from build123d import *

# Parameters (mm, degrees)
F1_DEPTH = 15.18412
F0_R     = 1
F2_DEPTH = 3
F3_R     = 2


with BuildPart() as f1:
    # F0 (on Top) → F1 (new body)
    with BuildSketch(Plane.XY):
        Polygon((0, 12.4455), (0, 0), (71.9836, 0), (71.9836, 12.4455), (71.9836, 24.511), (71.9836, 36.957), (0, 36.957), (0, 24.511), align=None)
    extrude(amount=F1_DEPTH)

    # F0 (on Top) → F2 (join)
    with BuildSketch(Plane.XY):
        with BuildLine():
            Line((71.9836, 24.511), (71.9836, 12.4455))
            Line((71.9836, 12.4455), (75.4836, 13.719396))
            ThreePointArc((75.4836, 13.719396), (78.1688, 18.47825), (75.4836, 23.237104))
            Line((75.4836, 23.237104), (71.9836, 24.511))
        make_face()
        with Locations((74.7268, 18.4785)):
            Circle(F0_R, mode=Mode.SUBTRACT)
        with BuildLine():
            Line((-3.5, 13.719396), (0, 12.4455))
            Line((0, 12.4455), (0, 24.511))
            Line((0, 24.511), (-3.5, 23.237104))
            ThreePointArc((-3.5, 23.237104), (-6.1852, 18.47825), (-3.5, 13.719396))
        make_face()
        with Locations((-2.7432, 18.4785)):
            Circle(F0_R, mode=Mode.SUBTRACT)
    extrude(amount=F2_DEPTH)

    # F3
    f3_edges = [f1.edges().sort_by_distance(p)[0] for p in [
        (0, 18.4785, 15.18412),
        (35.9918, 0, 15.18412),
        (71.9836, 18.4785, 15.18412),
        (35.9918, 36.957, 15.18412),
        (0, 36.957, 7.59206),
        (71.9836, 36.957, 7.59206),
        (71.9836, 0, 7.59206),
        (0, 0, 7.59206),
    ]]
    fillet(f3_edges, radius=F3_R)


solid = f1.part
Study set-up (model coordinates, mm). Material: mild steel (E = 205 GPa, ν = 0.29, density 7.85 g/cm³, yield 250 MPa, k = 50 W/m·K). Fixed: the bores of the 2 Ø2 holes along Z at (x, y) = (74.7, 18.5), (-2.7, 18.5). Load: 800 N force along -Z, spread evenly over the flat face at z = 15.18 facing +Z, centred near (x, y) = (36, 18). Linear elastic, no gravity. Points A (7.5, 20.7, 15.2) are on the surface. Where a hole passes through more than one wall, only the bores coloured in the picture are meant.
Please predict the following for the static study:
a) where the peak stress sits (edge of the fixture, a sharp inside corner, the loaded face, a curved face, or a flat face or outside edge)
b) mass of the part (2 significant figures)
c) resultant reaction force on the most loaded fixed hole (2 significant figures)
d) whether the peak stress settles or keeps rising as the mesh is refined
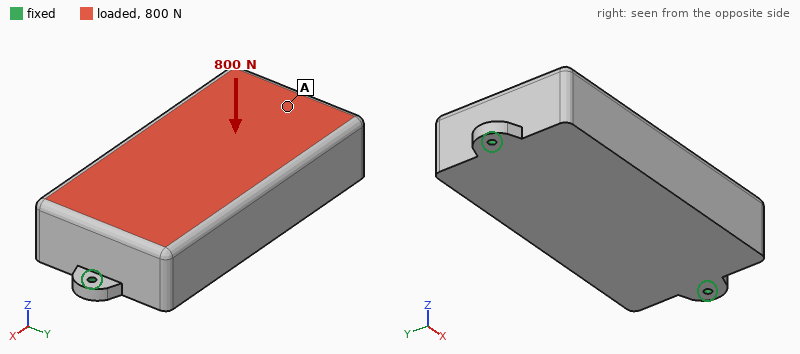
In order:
edge of the fixture
320 g
510 N
keeps rising
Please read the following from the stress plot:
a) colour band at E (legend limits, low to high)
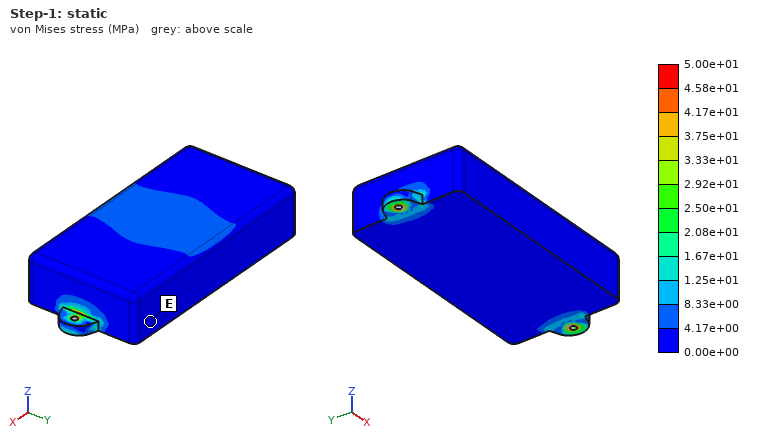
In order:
0.00e+00 to 4.17e+00 MPa
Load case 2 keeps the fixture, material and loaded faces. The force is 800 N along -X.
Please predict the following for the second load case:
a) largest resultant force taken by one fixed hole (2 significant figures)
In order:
430 N
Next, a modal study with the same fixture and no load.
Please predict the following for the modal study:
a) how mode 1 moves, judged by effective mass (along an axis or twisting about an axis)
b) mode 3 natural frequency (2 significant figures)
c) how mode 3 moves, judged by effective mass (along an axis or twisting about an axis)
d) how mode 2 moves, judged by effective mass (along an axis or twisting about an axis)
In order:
along Y
8000 Hz
along Y
along Z
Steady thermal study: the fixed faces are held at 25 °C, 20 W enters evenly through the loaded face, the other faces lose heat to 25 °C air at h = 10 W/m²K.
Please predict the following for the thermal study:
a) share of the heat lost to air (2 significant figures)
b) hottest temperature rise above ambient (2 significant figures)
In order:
11 %
40 K
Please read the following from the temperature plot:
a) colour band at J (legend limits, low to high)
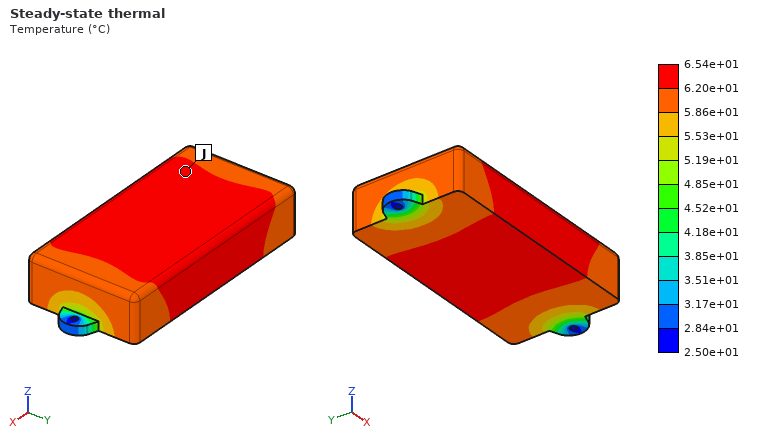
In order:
6.20e+01 to 6.54e+01 °C
